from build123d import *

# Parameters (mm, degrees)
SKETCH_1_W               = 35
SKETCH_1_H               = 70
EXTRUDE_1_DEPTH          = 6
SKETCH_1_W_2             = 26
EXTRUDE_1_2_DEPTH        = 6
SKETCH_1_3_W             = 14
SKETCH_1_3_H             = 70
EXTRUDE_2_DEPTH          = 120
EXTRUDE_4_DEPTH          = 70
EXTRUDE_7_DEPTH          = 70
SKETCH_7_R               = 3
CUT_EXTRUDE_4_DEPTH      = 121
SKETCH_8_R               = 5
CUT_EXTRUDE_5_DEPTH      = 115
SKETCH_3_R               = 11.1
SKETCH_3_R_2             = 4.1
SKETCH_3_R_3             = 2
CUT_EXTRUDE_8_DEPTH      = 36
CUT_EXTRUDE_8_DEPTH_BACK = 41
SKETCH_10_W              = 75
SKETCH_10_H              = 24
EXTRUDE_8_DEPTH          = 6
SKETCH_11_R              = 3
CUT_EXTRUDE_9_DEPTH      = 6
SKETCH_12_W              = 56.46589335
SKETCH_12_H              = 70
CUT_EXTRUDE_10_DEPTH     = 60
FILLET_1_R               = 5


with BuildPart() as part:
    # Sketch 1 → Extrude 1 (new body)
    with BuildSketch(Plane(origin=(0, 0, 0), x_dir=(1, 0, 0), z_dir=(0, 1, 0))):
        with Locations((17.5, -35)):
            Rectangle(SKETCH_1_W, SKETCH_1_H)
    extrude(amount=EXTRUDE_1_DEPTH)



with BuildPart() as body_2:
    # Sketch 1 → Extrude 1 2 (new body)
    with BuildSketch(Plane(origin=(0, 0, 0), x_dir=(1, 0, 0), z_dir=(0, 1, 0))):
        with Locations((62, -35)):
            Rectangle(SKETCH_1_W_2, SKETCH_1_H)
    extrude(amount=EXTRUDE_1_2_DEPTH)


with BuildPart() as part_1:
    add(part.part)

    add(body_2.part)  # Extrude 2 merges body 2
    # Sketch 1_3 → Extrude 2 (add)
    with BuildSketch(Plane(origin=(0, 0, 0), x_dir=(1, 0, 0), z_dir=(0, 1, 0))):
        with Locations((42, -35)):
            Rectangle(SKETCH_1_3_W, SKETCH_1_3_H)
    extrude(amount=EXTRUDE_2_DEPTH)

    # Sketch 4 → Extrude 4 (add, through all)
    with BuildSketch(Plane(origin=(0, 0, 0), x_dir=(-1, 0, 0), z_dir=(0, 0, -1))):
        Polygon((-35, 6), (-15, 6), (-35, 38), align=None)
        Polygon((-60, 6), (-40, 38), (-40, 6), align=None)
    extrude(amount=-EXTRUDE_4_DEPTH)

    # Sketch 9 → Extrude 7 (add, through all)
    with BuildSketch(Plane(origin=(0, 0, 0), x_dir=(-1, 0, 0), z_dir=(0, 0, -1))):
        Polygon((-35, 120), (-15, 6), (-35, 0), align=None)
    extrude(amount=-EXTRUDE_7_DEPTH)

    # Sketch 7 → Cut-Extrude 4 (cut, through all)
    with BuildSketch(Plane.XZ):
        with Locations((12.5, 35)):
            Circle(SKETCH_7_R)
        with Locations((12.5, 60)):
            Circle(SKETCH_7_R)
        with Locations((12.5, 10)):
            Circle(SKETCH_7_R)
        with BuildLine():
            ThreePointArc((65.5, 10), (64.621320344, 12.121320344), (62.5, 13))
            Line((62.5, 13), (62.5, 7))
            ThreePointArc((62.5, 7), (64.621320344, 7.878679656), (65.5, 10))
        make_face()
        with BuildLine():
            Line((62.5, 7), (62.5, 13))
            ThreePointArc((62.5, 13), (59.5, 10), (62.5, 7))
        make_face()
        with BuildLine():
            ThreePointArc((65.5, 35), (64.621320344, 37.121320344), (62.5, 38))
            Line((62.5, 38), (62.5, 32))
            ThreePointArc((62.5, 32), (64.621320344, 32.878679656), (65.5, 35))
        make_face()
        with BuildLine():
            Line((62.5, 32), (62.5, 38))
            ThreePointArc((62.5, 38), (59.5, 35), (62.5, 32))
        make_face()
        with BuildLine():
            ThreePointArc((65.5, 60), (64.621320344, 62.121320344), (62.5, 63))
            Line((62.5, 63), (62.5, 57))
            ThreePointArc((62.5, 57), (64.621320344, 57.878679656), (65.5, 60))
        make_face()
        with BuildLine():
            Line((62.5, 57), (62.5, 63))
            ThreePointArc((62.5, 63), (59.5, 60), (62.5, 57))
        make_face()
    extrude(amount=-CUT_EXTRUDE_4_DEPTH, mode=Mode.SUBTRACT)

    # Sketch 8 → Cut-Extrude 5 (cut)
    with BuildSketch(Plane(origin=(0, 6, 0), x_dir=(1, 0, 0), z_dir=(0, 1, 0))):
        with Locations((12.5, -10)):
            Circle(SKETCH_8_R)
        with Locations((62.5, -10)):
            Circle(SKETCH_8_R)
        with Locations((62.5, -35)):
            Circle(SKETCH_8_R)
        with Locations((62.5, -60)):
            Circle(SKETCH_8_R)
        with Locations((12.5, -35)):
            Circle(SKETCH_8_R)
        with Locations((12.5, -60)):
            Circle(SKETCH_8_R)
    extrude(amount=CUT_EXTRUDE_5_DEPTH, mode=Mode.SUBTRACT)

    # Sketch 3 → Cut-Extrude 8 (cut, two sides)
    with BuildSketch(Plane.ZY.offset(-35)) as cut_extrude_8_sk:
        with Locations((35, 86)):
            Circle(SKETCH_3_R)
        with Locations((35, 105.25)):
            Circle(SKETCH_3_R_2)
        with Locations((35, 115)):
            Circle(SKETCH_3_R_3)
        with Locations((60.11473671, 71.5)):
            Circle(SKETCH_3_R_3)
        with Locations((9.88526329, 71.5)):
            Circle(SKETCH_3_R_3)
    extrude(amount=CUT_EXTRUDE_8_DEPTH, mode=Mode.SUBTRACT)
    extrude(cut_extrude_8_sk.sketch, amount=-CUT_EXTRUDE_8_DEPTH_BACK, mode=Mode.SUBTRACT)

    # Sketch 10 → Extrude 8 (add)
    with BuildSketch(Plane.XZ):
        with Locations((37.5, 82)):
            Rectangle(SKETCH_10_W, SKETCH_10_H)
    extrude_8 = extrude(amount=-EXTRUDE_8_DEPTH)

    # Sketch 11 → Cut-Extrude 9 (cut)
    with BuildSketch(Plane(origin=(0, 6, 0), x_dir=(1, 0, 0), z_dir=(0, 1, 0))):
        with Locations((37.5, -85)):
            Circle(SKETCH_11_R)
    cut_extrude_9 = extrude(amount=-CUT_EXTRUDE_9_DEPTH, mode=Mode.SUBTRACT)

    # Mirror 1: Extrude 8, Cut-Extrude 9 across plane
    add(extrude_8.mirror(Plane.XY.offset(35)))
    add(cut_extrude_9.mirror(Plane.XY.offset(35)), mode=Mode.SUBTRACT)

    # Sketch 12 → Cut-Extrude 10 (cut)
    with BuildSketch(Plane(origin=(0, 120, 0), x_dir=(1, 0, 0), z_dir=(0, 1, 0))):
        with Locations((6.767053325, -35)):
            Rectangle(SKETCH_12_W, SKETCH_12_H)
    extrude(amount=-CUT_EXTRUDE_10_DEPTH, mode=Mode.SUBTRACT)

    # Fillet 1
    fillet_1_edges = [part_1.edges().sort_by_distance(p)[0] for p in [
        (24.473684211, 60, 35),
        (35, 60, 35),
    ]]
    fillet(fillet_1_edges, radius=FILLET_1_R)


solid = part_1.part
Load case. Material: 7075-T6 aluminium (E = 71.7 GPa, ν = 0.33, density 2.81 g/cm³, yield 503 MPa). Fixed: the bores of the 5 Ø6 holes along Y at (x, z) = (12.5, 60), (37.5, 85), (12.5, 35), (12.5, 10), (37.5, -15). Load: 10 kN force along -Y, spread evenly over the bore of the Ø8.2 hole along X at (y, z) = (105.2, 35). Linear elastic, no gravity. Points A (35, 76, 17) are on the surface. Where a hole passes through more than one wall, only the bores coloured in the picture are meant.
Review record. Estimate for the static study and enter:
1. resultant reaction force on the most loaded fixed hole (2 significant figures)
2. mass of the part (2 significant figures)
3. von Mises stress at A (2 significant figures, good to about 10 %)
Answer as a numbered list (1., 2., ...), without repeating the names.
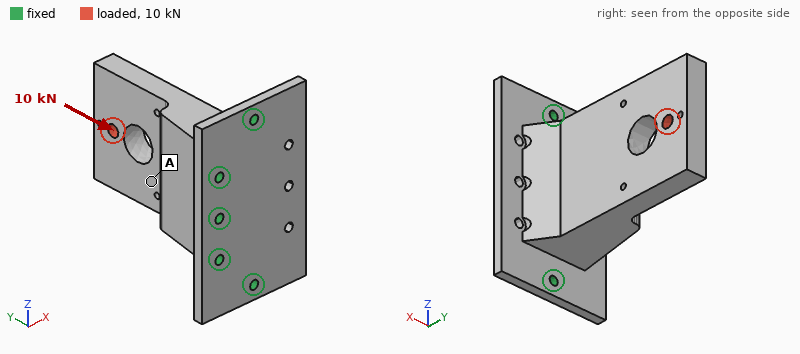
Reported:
1. 4.5 kN
2. 620 g
3. 25 MPa
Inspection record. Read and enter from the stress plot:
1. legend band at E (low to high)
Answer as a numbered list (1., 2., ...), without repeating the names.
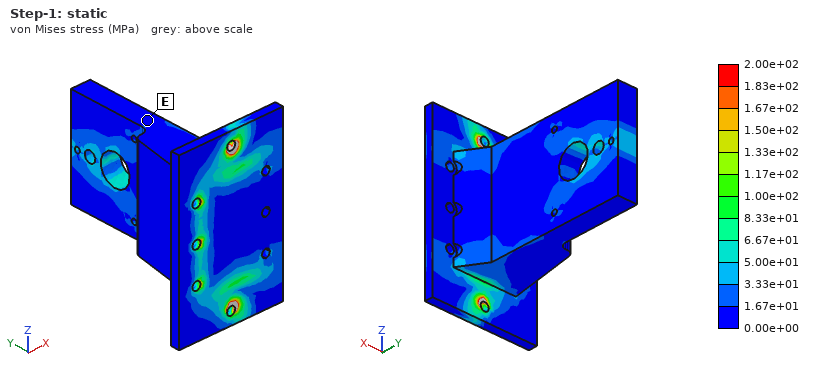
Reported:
1. 0.00e+00 to 1.67e+01 MPa
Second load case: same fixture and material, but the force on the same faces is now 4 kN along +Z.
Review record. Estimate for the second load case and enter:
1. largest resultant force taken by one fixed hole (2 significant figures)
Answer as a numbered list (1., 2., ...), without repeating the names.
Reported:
1. 5.0 kN
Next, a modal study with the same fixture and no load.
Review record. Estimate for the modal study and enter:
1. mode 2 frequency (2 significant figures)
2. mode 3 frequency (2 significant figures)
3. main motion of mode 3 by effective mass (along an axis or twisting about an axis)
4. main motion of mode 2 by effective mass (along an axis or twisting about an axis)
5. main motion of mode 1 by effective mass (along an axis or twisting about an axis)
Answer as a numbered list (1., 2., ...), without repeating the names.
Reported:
1. 2600 Hz
2. 3600 Hz
3. along Y
4. along Z
5. along X
